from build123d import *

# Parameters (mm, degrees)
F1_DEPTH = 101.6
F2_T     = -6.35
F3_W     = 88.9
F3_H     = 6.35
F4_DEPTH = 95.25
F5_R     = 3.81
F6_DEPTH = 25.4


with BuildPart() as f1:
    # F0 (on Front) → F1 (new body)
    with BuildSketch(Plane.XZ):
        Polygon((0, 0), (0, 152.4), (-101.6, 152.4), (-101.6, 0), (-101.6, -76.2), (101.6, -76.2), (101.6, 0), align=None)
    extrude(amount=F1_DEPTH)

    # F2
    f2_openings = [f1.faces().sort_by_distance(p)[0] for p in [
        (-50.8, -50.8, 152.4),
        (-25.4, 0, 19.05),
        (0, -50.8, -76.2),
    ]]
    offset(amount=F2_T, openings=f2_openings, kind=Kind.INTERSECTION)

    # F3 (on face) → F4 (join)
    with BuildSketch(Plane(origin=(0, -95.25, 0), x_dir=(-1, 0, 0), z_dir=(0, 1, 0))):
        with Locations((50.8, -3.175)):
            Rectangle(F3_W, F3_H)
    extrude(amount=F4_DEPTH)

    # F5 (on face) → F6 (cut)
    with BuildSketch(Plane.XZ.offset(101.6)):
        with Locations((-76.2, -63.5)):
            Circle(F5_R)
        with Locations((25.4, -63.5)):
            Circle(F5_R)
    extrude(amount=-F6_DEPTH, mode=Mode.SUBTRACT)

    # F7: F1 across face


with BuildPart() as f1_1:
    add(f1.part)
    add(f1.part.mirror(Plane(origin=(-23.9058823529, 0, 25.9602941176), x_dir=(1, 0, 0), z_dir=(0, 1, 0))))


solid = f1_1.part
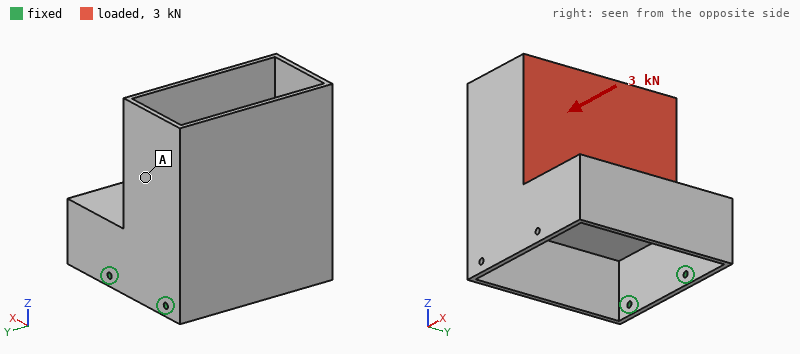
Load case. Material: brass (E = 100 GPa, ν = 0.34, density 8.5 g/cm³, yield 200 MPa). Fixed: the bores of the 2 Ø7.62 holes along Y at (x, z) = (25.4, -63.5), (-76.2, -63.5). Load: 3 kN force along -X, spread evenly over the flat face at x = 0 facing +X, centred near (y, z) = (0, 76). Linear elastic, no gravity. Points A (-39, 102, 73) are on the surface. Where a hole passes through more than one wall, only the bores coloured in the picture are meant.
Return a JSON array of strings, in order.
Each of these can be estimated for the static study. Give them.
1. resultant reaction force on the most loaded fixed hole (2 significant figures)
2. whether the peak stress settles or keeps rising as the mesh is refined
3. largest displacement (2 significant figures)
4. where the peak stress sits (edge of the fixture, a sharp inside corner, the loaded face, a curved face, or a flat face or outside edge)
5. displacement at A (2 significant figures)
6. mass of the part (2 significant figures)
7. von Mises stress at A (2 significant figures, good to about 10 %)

["4.9 kN", "keeps rising", "1.1 mm", "edge of the fixture", "0.30 mm", "10.0 kg", "10 MPa"]
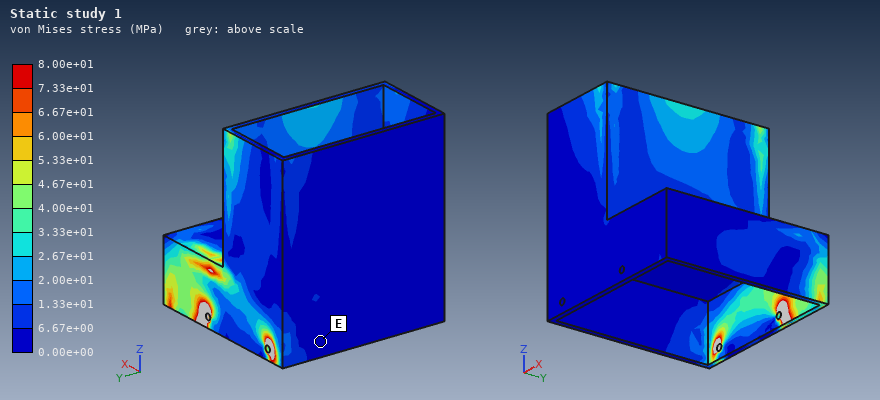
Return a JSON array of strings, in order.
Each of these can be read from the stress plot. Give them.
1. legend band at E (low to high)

["0.00e+00 to 6.67e+00 MPa"]
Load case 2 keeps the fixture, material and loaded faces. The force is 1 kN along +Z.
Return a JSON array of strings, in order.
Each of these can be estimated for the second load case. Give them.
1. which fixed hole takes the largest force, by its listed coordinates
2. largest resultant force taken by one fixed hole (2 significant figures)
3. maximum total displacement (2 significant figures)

["(25.4, -63.5)", "770 N", "2.1 mm"]
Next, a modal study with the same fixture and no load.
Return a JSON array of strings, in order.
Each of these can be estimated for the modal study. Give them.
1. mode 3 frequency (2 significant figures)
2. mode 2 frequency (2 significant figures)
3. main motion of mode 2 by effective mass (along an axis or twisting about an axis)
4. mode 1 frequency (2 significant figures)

["190 Hz", "110 Hz", "along X", "37 Hz"]
